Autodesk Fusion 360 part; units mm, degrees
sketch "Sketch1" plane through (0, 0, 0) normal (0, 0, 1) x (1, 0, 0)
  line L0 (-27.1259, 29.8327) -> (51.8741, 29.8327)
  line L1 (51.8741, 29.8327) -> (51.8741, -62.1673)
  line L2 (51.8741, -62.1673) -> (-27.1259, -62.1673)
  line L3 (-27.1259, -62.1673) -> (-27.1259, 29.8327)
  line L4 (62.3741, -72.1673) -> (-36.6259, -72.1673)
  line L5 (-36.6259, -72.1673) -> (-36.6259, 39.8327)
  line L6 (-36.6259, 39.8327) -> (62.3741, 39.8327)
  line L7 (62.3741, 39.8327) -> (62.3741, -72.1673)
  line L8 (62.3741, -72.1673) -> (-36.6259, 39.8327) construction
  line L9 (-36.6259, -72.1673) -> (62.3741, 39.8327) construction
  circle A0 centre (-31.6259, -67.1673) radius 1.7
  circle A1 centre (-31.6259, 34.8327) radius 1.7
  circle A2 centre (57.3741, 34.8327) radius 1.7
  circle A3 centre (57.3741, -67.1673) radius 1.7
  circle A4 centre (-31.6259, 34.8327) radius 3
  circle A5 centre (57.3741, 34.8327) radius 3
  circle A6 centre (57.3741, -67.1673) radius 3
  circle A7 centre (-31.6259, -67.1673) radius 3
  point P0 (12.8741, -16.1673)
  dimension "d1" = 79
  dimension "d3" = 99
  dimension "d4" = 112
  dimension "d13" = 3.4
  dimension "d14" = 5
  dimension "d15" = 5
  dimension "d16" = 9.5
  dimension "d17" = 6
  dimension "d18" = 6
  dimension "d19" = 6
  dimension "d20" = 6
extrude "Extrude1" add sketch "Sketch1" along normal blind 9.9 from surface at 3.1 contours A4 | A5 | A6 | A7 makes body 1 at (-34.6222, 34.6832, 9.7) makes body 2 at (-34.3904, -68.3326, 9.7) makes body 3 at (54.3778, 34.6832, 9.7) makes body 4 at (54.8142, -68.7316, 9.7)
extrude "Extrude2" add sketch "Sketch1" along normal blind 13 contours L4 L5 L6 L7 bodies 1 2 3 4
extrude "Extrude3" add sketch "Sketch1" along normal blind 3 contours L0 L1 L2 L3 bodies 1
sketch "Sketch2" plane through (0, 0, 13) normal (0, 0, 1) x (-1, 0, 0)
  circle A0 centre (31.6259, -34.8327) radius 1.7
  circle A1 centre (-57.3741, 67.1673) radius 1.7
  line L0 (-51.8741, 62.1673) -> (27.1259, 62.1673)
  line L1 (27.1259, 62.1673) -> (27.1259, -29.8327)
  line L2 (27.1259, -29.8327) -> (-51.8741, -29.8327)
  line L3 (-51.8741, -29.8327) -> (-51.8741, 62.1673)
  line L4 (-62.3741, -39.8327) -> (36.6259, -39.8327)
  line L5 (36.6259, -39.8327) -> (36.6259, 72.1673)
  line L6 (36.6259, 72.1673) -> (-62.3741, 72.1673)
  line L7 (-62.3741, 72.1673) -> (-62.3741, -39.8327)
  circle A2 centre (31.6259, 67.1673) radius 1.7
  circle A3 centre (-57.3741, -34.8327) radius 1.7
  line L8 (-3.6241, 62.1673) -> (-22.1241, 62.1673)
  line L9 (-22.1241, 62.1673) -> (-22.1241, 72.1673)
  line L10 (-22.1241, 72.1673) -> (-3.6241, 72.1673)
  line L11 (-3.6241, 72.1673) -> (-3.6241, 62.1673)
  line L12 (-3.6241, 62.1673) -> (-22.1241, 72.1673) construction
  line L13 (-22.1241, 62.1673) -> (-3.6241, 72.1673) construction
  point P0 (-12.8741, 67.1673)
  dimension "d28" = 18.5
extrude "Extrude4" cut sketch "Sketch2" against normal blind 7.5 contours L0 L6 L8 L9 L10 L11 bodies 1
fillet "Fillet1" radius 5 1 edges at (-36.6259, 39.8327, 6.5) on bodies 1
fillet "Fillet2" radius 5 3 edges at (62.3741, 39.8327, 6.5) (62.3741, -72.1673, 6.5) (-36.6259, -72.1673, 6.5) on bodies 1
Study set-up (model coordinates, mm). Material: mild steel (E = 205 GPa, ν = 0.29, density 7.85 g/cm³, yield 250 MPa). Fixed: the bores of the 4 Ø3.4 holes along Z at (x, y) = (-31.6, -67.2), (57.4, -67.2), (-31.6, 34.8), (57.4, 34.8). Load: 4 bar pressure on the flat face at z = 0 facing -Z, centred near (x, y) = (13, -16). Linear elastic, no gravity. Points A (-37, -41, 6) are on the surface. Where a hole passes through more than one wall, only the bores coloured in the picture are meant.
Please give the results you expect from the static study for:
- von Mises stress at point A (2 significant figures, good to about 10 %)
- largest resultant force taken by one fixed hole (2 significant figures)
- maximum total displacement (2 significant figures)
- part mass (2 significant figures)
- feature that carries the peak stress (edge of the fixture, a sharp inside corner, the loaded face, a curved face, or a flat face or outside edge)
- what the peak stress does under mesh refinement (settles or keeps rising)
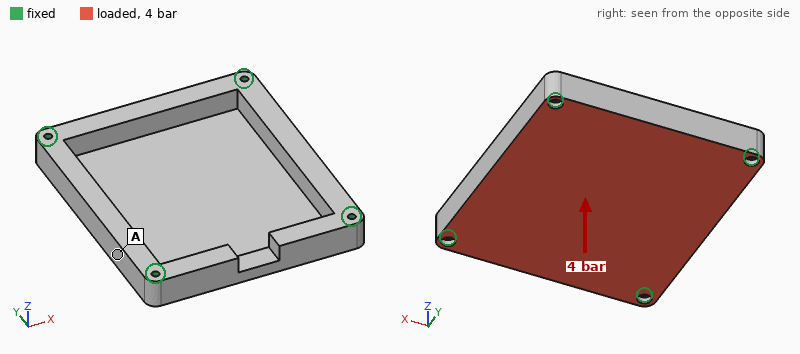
12 MPa
1.9 kN
89 µm
540 g
edge of the fixture
keeps rising
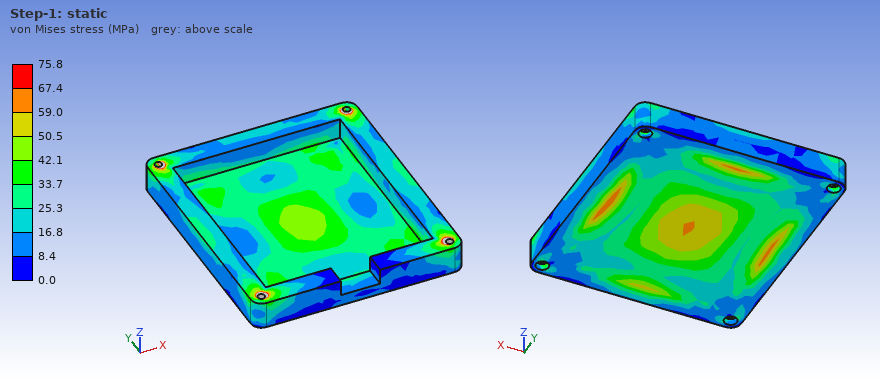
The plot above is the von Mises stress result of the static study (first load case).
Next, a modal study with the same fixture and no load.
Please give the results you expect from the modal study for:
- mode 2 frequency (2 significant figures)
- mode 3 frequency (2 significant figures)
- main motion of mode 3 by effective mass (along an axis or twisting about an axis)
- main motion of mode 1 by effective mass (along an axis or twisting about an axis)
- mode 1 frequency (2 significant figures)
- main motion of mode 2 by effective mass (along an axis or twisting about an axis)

4700 Hz
5000 Hz
twisting about X
along Z
2800 Hz
twisting about Y
